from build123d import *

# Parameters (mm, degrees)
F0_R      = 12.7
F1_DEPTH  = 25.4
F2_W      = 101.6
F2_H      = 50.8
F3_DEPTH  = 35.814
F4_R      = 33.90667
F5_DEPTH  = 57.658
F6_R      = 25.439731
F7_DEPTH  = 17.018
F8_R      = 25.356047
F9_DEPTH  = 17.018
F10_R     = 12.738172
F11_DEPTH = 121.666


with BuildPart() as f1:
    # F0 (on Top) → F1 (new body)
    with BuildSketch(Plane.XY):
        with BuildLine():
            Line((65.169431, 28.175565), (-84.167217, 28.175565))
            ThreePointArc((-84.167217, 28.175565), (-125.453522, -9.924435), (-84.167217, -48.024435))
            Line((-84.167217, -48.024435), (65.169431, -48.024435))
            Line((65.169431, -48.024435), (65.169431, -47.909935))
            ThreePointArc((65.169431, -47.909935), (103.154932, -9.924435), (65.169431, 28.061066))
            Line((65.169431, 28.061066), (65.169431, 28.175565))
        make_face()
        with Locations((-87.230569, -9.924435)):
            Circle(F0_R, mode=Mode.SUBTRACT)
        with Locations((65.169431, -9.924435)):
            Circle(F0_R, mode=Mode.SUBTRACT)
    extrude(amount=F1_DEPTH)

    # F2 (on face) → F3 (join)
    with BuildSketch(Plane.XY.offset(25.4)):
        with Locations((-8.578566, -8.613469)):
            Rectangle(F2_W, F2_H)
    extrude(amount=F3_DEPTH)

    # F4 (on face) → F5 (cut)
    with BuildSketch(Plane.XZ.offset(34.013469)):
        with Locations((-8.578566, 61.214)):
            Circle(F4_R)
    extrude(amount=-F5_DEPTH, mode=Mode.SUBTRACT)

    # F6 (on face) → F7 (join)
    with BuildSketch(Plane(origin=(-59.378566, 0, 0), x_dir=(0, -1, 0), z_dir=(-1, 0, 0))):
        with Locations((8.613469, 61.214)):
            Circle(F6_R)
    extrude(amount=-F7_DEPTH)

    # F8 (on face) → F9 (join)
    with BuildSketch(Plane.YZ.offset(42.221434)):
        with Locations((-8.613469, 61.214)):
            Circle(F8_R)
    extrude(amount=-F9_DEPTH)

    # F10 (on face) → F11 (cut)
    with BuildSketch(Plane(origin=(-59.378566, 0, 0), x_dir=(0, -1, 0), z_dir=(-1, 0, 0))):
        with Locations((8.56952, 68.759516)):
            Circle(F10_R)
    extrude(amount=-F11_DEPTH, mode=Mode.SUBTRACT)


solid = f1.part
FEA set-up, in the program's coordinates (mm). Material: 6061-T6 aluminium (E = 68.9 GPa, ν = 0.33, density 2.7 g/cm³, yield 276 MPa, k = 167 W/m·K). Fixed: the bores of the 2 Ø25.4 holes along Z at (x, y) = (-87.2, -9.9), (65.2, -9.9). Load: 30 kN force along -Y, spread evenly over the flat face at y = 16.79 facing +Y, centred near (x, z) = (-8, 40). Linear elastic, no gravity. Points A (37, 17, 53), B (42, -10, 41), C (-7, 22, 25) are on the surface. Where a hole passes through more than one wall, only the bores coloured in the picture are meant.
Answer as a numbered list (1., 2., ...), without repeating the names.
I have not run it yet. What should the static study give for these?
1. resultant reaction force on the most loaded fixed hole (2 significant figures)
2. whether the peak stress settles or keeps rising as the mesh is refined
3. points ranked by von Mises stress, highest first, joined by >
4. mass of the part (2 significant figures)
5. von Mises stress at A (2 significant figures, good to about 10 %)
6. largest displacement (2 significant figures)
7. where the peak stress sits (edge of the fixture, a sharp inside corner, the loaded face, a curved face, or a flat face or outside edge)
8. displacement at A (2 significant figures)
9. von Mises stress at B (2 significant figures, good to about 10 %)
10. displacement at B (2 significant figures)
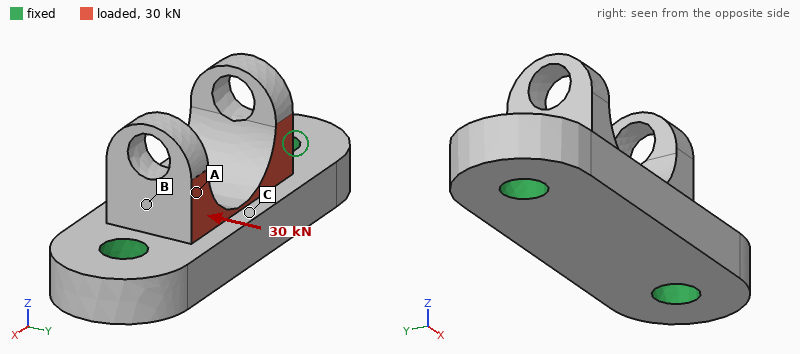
1. 16 kN
2. keeps rising
3. B > A > C
4. 1.3 kg
5. 15 MPa
6. 0.11 mm
7. edge of the fixture
8. 0.076 mm
9. 22 MPa
10. 0.047 mm
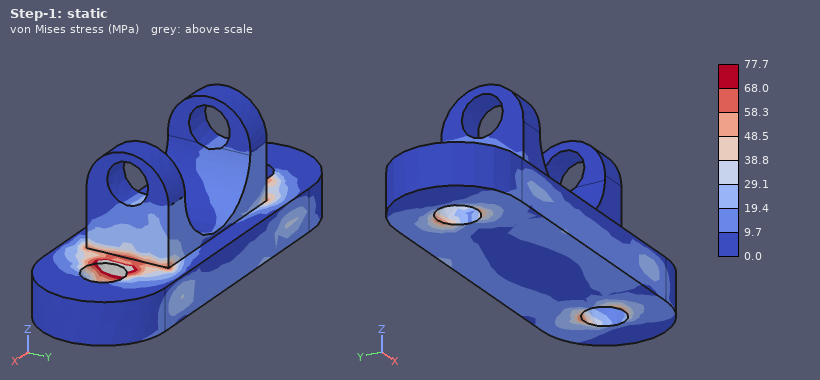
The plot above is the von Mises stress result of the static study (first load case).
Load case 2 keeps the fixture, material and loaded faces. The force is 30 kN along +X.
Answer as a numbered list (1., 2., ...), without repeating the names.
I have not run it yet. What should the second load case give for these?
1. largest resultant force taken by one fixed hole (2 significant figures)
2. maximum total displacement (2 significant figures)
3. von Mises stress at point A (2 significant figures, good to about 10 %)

1. 17 kN
2. 70 µm
3. 45 MPa
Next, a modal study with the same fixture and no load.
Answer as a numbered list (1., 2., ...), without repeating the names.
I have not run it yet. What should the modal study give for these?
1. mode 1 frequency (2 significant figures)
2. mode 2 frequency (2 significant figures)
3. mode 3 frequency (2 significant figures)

1. 4400 Hz
2. 4500 Hz
3. 6500 Hz
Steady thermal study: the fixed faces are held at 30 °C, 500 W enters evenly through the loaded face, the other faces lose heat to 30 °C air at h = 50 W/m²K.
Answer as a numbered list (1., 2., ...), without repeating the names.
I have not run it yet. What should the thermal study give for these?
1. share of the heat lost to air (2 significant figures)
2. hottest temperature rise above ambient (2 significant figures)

1. 11 %
2. 63 K
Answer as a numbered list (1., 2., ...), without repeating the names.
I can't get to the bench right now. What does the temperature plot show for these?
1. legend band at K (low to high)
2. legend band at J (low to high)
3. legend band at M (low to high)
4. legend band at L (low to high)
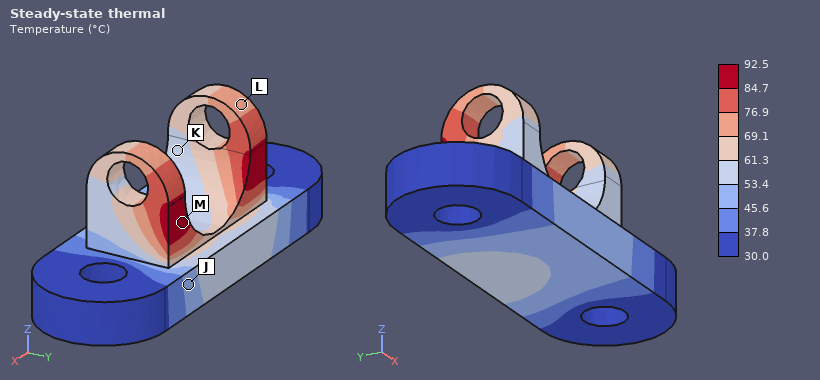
1. 53.4 to 61.3 °C
2. 45.6 to 53.4 °C
3. 84.7 to 92.5 °C
4. 69.1 to 76.9 °C
